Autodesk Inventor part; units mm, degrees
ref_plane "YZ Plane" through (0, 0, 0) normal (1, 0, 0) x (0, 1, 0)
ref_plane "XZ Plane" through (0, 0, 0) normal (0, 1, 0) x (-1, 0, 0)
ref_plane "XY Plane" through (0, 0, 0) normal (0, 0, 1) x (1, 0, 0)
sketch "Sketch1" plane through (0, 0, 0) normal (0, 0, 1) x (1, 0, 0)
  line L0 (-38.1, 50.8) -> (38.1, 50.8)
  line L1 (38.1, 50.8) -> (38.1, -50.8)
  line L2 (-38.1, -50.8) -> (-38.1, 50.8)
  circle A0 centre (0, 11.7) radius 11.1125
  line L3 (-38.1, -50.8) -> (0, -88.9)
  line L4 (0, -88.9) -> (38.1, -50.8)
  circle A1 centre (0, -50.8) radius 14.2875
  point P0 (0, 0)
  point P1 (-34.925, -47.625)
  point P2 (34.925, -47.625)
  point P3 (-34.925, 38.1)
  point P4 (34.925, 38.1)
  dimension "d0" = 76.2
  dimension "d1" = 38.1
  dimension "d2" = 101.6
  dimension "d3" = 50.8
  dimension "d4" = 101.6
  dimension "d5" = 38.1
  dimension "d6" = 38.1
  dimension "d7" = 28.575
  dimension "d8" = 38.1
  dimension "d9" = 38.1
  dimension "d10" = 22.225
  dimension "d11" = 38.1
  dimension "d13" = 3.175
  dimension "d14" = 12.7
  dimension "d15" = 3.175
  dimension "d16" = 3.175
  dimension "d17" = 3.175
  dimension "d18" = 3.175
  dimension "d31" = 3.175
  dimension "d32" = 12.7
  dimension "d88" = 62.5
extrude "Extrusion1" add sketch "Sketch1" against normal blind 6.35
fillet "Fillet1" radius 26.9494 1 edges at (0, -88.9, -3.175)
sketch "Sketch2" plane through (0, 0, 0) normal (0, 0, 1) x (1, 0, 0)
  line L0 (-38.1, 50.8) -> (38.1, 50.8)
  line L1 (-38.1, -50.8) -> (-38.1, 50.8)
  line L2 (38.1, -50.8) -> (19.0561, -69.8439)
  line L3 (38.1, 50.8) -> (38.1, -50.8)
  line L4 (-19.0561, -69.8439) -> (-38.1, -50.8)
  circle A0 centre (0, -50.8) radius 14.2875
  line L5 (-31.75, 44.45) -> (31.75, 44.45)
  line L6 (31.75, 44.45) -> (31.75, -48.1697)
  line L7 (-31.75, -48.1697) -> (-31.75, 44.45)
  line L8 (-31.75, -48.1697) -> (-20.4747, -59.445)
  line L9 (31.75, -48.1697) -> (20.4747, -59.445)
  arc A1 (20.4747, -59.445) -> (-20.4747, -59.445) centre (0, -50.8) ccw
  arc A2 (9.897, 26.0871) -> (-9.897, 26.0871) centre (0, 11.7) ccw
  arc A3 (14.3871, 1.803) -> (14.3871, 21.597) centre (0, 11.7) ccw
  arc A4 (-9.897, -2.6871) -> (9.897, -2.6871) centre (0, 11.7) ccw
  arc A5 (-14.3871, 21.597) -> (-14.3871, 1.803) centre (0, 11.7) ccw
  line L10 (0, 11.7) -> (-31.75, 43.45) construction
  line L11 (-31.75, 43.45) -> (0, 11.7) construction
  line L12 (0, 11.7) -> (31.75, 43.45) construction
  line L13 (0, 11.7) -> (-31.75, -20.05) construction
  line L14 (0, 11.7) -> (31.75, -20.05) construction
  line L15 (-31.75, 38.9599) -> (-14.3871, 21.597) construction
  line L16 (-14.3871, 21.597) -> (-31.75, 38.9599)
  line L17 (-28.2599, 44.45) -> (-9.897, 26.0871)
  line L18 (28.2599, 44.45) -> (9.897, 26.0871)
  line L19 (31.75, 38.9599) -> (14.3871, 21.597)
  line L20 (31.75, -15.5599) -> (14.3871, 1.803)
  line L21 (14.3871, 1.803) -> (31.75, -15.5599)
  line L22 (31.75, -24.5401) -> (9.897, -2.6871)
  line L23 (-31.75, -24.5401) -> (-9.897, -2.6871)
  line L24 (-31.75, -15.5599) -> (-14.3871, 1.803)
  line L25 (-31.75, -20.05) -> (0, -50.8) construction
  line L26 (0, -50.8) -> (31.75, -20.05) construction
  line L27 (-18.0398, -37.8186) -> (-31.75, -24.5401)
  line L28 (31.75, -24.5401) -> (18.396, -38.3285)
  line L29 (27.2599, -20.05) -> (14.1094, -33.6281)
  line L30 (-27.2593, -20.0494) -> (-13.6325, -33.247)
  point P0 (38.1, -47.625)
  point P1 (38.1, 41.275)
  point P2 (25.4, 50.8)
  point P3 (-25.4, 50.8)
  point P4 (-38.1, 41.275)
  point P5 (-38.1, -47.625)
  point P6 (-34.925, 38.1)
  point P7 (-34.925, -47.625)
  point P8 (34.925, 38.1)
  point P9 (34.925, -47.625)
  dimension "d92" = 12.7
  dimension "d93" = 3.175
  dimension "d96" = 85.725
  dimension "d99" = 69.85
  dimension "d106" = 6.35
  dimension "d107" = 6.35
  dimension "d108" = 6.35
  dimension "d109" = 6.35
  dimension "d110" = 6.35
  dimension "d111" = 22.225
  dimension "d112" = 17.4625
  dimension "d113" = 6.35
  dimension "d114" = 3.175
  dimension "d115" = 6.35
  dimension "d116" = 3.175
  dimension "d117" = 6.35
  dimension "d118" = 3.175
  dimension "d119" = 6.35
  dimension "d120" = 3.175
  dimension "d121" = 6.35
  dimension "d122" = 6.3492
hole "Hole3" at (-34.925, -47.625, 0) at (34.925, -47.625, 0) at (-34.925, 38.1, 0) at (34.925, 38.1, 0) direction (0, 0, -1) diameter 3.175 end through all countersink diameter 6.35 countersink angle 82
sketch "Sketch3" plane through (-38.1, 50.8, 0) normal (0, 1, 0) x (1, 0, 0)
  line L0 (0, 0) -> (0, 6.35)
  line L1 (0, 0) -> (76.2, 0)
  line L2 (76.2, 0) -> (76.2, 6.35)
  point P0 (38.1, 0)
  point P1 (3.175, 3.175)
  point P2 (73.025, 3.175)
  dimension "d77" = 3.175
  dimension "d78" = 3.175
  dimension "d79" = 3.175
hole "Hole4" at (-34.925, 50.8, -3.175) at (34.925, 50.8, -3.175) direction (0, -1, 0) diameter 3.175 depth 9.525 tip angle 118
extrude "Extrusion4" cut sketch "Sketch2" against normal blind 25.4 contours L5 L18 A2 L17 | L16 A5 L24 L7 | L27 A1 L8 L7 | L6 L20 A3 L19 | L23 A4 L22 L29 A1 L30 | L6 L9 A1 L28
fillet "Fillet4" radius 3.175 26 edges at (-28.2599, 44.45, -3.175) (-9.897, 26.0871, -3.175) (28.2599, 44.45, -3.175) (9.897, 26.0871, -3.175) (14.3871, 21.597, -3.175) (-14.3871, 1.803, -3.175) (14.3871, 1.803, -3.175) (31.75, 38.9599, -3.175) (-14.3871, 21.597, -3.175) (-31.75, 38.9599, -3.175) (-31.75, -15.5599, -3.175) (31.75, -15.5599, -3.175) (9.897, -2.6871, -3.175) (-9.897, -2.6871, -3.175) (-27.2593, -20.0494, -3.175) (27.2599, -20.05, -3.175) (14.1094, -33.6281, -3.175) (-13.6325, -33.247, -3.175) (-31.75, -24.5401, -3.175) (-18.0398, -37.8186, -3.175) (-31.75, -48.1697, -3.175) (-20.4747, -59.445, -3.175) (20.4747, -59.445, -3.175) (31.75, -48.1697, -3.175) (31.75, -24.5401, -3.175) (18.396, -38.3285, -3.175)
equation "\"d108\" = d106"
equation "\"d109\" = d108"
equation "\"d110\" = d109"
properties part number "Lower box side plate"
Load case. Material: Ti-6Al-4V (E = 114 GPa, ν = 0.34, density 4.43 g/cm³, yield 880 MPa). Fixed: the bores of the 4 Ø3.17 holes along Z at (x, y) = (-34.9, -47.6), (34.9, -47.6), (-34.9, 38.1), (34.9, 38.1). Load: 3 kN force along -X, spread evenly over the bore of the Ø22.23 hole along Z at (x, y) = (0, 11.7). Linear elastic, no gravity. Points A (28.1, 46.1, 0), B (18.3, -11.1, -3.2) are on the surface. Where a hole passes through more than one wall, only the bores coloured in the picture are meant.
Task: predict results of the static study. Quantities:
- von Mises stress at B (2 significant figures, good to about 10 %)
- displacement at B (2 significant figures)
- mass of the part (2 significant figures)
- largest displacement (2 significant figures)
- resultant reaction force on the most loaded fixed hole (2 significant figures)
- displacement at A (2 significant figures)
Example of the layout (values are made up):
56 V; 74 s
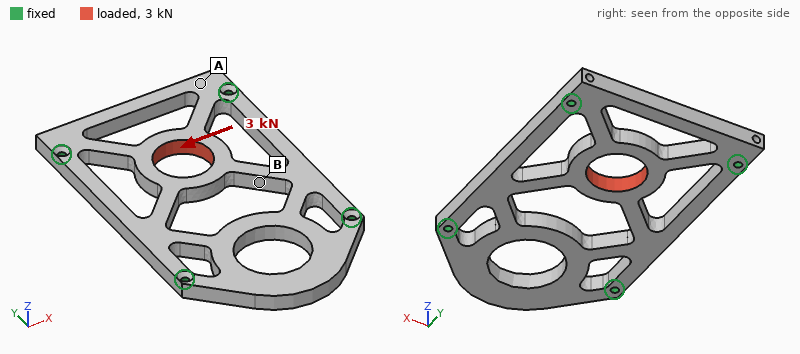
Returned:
21 MPa; 25 µm; 130 g; 32 µm; 1.1 kN; 4.8 µm
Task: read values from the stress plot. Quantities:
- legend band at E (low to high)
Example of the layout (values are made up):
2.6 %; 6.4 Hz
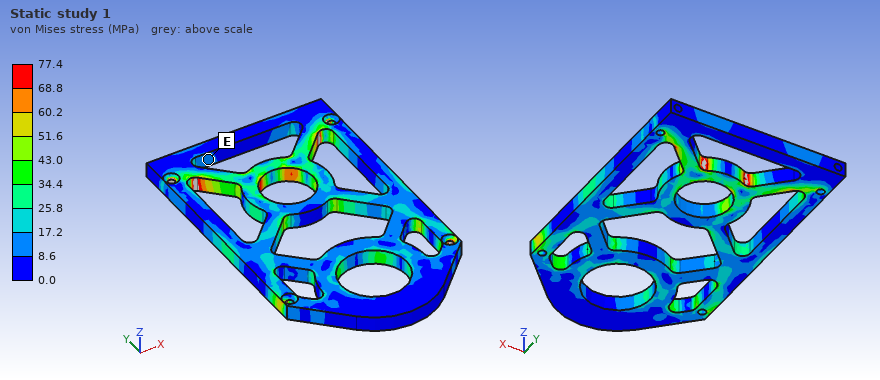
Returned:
8.6 to 17.2 MPa
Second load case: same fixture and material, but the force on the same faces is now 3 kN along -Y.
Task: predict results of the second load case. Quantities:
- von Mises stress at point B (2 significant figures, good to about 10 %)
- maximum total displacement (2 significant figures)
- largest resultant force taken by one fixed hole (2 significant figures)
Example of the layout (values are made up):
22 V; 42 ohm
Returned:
26 MPa; 22 µm; 1.1 kN
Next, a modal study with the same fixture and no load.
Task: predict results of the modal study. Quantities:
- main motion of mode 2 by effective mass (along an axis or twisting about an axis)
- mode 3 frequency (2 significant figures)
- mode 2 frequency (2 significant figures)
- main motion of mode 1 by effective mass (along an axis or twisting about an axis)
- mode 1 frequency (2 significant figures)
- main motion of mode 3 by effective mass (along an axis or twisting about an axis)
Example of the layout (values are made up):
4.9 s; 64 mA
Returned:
along Z; 4200 Hz; 3000 Hz; along Z; 2600 Hz; twisting about Y
